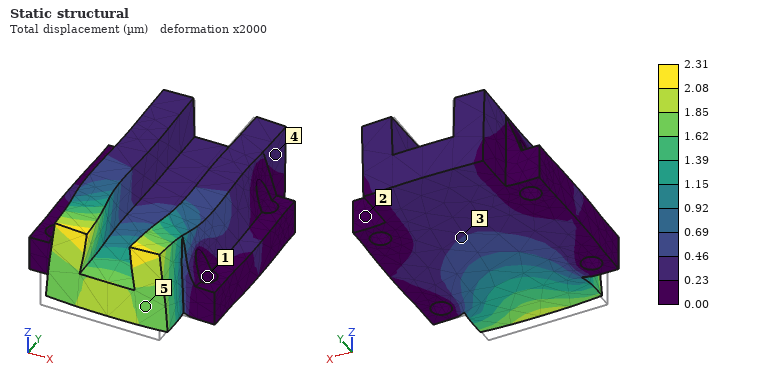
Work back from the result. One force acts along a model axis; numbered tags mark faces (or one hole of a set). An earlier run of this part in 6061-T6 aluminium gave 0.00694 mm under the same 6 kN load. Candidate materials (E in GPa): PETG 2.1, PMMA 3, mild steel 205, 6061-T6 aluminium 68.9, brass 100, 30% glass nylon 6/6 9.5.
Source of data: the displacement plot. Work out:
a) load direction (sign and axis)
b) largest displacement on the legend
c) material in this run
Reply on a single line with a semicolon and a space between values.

+Y; 2.31 µm; mild steel
